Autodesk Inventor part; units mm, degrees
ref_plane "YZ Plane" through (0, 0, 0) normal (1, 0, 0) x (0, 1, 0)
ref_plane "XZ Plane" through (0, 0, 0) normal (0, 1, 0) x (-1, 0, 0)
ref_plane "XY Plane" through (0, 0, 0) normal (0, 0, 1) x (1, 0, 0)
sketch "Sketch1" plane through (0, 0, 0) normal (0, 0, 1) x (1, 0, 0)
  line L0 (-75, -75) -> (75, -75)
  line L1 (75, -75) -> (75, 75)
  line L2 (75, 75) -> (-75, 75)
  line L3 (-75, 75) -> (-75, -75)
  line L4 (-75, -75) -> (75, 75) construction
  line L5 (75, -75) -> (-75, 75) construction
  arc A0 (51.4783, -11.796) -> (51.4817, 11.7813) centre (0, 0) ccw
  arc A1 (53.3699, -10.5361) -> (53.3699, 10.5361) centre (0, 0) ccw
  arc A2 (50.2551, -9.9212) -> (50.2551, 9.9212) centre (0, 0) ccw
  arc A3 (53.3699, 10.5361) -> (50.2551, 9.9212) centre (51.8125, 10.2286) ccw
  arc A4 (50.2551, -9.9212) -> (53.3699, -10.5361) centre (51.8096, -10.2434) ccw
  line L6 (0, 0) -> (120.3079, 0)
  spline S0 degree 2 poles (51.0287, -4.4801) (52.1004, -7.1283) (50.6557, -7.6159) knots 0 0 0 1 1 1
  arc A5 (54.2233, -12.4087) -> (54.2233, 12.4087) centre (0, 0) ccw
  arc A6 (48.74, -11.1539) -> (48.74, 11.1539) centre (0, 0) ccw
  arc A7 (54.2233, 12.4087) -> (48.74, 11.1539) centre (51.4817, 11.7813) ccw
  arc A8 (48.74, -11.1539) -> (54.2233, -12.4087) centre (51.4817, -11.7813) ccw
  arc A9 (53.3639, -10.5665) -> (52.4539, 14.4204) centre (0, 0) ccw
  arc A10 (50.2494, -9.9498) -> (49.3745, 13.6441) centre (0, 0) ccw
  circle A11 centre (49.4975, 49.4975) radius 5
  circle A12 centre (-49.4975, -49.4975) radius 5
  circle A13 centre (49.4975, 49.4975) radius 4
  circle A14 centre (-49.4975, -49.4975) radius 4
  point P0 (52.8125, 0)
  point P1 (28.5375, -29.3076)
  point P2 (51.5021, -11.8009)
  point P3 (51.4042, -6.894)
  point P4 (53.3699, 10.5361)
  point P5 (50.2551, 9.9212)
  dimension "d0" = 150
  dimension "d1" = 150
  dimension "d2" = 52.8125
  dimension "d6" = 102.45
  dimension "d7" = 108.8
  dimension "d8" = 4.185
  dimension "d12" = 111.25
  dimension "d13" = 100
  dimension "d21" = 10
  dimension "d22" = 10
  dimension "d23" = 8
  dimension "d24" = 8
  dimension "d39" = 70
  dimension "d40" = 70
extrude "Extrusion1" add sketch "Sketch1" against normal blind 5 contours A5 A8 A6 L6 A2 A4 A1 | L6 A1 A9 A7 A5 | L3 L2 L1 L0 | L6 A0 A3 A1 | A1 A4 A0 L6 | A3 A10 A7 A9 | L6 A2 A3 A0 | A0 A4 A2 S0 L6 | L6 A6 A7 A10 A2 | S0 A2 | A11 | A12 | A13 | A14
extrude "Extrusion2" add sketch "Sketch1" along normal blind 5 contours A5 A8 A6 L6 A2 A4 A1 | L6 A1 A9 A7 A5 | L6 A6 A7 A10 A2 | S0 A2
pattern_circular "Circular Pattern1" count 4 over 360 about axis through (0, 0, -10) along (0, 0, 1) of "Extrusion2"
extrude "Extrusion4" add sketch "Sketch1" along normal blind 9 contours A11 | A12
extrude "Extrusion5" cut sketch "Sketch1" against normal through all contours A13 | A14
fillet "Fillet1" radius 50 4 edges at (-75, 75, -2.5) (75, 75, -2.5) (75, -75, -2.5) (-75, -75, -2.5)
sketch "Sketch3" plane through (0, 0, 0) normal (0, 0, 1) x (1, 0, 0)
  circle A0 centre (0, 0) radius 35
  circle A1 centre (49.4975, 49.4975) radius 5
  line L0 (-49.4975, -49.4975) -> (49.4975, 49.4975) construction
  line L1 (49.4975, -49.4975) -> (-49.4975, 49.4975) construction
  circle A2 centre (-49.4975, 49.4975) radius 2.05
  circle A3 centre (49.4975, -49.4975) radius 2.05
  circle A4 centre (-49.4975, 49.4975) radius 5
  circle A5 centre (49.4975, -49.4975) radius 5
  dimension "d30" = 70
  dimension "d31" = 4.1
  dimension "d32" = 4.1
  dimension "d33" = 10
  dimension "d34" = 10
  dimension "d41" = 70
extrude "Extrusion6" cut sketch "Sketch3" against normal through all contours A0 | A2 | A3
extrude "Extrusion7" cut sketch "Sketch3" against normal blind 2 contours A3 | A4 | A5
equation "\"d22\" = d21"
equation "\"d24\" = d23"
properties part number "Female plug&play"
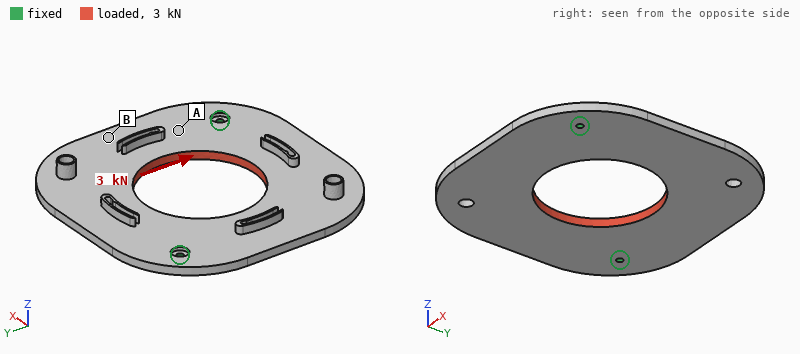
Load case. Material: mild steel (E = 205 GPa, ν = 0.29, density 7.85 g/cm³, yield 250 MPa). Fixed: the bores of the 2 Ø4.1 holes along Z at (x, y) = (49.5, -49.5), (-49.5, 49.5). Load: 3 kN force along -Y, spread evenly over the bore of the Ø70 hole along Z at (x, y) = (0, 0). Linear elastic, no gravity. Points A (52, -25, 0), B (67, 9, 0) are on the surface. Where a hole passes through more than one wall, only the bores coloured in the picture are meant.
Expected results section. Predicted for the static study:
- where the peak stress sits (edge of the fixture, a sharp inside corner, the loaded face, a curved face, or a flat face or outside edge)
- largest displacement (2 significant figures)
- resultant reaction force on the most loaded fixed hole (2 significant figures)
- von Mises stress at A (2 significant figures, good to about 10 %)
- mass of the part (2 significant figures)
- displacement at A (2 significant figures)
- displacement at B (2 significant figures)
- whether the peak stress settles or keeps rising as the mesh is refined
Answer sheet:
edge of the fixture
19 µm
1.5 kN
6.3 MPa
660 g
5.8 µm
13 µm
keeps rising
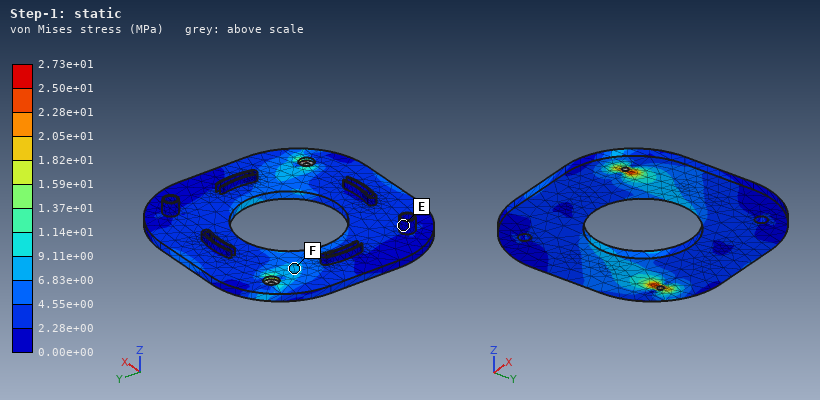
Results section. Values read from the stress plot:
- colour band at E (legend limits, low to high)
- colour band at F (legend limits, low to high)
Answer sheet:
0.00e+00 to 2.28e+00 MPa
6.83e+00 to 9.11e+00 MPa
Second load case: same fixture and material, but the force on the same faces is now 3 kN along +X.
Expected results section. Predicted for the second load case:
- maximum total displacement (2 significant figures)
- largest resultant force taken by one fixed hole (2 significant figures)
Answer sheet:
19 µm
1.5 kN
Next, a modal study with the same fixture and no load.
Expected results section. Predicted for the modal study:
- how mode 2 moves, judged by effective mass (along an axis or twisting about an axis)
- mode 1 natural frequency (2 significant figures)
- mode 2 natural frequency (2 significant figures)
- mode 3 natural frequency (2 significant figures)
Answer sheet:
along Z
350 Hz
520 Hz
1300 Hz
